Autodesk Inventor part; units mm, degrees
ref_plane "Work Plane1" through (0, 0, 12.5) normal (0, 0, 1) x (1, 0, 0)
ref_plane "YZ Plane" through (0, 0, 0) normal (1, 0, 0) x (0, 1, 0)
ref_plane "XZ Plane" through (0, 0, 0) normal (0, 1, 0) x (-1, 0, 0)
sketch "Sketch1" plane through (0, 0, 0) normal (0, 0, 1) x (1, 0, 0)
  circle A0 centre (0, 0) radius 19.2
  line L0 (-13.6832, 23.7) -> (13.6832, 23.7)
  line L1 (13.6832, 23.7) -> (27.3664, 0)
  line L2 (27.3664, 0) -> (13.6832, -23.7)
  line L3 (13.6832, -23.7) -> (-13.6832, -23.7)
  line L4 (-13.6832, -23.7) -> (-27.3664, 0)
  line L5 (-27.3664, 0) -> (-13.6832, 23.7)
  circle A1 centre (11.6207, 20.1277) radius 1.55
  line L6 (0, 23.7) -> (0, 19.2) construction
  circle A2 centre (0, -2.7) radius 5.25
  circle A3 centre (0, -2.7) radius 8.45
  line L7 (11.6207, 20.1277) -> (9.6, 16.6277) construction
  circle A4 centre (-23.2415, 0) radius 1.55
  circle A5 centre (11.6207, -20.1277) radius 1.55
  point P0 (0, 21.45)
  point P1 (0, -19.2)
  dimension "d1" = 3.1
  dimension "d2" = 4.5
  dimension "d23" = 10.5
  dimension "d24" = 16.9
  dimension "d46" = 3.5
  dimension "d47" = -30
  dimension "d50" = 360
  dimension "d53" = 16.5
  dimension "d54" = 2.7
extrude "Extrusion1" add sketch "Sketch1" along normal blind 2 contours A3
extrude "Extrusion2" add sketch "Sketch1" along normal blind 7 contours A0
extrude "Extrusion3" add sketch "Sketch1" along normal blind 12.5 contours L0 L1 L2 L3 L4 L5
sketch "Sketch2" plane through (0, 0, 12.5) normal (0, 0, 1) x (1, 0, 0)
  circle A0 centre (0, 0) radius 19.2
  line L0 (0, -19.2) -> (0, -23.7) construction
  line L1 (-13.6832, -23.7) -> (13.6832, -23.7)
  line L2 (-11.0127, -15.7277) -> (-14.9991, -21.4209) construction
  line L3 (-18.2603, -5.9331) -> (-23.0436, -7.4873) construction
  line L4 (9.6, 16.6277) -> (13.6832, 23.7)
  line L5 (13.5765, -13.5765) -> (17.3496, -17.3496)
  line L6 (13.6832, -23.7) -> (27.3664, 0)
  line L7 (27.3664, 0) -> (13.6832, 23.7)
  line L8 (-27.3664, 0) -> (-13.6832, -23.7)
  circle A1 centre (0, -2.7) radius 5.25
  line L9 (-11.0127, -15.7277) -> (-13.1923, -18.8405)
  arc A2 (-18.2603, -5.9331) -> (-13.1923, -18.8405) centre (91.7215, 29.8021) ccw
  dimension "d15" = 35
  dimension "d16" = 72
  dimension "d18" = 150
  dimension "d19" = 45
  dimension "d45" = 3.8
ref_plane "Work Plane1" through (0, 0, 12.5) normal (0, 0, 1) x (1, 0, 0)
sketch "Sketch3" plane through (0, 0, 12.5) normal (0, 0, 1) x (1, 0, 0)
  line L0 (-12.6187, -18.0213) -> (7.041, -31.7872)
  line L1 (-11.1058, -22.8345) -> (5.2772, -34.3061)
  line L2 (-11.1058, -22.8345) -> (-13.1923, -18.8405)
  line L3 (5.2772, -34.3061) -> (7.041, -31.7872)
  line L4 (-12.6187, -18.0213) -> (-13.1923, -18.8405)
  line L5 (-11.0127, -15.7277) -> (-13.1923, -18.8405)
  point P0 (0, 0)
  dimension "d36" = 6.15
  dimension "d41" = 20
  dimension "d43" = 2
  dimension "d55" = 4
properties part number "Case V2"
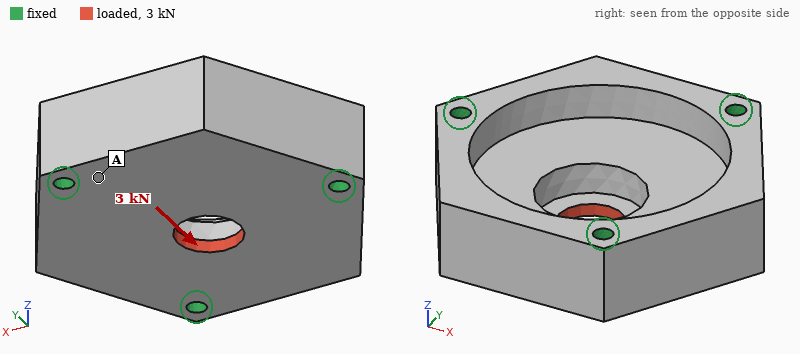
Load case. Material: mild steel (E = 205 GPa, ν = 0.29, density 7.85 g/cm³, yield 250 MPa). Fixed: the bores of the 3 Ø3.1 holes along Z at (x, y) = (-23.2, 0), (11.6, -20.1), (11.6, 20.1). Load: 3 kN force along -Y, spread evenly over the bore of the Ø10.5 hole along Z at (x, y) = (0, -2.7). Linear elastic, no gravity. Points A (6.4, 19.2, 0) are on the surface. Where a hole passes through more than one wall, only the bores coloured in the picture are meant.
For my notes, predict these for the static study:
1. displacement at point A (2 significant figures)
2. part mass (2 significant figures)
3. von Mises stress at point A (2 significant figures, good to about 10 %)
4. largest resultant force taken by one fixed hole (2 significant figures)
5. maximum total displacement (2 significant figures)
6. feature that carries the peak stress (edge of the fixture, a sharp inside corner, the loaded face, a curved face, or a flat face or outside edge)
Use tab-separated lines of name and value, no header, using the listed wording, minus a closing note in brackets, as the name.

displacement at point A	0.58 µm
part mass	130 g
von Mises stress at point A	12 MPa
largest resultant force taken by one fixed hole	1.1 kN
maximum total displacement	3.4 µm
feature that carries the peak stress	the loaded face
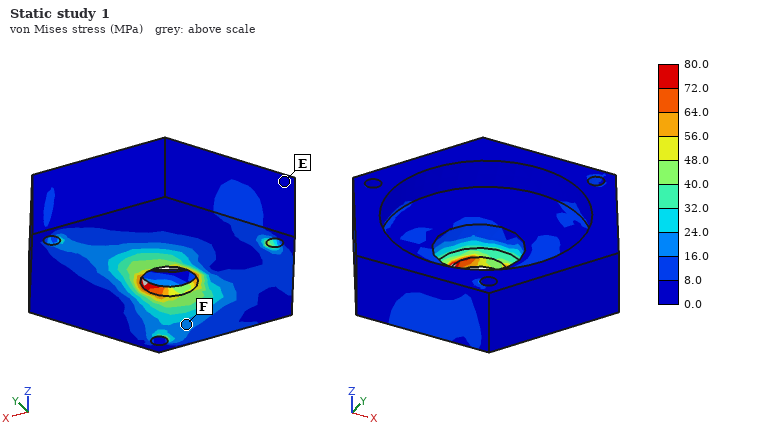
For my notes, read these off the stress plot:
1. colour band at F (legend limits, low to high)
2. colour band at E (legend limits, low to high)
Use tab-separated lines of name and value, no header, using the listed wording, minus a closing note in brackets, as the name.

colour band at F	16.0 to 24.0 MPa
colour band at E	0.0 to 8.0 MPa
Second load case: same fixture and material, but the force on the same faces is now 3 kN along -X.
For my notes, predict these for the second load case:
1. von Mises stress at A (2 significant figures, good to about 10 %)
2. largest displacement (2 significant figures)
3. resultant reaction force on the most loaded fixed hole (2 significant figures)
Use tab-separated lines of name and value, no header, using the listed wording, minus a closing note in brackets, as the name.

von Mises stress at A	8.1 MPa
largest displacement	3.5 µm
resultant reaction force on the most loaded fixed hole	1.1 kN
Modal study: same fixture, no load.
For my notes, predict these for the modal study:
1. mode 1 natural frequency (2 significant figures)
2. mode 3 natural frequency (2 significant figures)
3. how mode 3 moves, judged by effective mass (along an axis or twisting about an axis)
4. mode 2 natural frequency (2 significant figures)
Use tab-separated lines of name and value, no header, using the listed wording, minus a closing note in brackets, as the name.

mode 1 natural frequency	18 kHz
mode 3 natural frequency	20 kHz
how mode 3 moves, judged by effective mass	along Z
mode 2 natural frequency	18 kHz
